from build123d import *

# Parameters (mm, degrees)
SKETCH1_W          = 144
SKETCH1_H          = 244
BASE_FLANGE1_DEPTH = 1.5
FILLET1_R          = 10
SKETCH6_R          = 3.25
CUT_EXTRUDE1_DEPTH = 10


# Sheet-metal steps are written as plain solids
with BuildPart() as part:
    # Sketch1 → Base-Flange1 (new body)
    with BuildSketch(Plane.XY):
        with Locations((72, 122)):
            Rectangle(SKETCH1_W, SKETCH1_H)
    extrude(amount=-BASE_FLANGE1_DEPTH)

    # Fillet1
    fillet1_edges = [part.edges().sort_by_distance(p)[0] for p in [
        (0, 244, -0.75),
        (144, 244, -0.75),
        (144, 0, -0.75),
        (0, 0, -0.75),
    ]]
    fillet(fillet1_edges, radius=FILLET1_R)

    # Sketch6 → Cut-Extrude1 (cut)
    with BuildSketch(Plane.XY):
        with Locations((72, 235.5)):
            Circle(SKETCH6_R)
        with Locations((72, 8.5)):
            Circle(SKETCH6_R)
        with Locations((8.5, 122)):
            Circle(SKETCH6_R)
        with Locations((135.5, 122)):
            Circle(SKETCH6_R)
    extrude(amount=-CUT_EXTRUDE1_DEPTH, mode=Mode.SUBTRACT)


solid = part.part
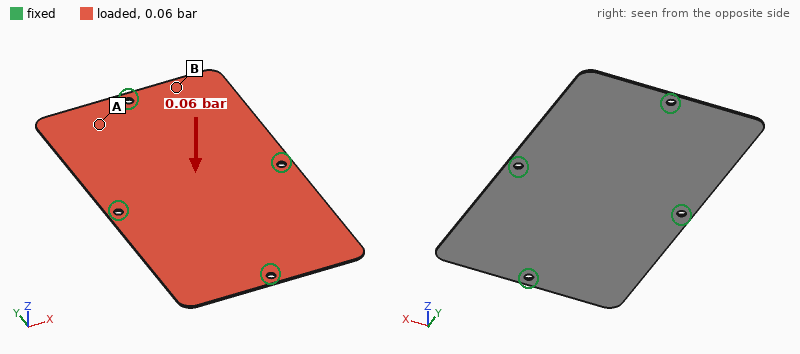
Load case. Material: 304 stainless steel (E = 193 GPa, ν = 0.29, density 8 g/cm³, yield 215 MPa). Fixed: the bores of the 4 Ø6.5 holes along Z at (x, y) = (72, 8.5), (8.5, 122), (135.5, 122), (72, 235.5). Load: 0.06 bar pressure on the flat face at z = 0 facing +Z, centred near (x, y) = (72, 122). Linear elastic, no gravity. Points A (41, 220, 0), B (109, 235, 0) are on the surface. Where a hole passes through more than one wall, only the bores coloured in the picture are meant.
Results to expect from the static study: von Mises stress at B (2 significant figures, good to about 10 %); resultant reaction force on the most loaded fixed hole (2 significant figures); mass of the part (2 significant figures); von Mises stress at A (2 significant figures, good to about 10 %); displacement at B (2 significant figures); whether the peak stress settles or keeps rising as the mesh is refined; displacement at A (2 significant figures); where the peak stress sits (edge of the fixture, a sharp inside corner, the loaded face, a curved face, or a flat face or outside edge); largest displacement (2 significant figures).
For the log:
4.9 MPa
53 N
420 g
9.5 MPa
0.085 mm
keeps rising
0.080 mm
edge of the fixture
0.21 mm
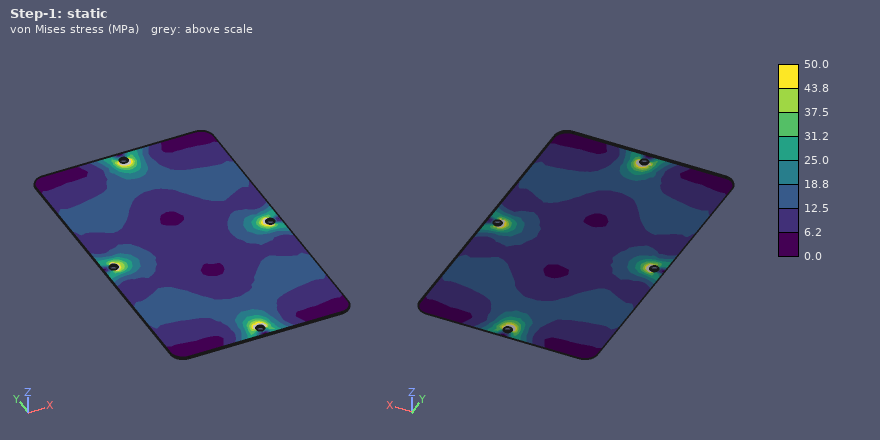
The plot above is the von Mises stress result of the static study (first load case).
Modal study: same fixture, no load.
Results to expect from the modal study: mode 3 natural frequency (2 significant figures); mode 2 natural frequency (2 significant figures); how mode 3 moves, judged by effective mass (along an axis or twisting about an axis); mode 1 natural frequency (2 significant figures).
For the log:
310 Hz
280 Hz
twisting about X
280 Hz
